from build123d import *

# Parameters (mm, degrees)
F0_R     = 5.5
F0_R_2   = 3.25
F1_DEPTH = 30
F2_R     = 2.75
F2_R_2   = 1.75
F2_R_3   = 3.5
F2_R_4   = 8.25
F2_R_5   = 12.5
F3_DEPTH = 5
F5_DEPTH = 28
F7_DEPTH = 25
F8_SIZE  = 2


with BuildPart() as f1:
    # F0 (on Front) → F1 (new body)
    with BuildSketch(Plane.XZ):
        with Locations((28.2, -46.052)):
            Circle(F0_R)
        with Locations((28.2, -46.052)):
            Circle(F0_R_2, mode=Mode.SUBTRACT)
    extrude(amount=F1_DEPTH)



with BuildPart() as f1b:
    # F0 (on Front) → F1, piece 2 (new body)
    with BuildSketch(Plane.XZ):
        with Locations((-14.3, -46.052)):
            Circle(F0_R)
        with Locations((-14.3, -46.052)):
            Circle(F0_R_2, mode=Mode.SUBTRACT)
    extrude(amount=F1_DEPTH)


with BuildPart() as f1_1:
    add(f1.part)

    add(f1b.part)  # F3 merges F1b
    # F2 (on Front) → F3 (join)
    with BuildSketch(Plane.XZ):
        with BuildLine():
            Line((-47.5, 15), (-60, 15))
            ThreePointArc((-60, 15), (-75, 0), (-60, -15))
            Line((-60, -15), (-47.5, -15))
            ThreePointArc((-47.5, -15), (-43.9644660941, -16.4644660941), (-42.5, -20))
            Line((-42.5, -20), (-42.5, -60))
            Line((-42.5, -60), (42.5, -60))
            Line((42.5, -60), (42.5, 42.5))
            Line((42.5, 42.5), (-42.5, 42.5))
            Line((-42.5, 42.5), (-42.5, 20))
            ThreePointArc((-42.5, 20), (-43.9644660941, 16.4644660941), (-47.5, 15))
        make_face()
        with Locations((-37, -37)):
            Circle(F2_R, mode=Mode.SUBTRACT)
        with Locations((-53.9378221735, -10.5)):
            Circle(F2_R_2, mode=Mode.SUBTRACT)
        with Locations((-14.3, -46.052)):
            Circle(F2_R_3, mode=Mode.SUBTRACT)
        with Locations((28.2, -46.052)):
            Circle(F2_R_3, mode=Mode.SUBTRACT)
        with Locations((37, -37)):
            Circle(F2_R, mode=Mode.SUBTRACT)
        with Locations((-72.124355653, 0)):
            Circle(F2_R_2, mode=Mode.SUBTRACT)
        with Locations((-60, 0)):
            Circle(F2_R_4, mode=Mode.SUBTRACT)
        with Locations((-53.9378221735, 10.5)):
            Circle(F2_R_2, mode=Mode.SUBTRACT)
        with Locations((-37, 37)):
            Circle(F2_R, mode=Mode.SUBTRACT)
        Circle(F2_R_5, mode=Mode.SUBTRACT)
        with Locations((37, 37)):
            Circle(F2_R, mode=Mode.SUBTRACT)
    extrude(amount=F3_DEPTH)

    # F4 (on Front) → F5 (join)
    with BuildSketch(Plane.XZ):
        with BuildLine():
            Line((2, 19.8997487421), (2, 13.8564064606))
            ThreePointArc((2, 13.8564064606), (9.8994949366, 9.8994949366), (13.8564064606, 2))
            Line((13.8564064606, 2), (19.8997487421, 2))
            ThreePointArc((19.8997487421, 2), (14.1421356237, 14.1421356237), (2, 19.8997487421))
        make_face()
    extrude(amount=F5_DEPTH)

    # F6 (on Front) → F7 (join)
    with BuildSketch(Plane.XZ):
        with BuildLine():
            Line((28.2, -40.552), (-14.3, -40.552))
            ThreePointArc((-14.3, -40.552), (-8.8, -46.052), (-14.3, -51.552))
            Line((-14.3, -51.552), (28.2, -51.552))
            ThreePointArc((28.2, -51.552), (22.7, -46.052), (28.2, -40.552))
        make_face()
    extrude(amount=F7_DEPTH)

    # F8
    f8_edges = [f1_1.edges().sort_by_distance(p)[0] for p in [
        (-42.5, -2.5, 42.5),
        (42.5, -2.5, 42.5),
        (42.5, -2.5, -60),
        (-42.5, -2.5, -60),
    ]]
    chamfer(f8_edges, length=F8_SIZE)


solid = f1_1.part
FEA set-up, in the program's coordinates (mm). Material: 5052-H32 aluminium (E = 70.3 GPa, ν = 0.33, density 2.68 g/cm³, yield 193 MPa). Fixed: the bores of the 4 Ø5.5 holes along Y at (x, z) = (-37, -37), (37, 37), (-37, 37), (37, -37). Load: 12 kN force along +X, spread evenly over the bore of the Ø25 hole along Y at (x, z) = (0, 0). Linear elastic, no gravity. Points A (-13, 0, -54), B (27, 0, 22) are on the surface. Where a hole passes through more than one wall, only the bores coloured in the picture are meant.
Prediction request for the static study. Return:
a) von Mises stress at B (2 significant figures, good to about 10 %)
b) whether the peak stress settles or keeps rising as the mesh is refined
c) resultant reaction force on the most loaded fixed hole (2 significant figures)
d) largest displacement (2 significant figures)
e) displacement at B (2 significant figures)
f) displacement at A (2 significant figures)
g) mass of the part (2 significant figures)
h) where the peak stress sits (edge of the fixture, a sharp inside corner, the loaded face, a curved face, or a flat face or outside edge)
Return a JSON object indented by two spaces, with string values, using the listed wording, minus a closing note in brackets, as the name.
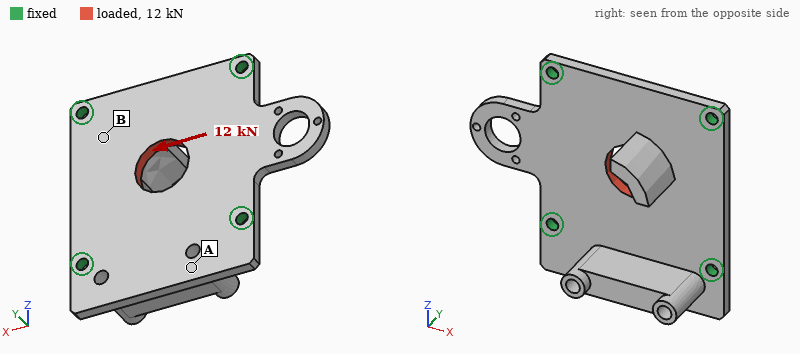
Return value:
{
  "von Mises stress at B": "30 MPa",
  "whether the peak stress settles or keeps rising as the mesh is refined": "keeps rising",
  "resultant reaction force on the most loaded fixed hole": "3.4 kN",
  "largest displacement": "27 µm",
  "displacement at B": "13 µm",
  "displacement at A": "5.0 µm",
  "mass of the part": "150 g",
  "where the peak stress sits": "edge of the fixture"
}
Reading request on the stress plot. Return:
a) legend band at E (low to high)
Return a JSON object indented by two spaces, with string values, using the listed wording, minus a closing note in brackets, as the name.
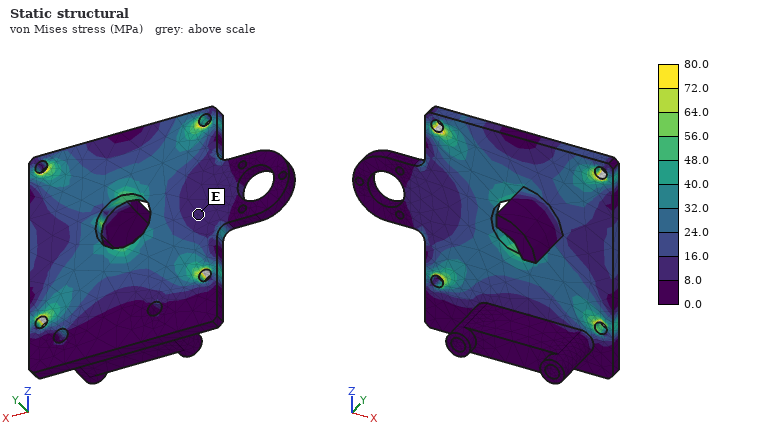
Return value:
{
  "legend band at E": "8.0 to 16.0 MPa"
}
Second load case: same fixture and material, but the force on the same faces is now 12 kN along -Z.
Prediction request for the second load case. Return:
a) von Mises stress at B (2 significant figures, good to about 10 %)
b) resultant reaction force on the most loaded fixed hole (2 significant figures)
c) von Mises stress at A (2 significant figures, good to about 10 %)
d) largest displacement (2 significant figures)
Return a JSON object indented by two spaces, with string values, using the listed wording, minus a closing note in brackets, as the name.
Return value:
{
  "von Mises stress at B": "28 MPa",
  "resultant reaction force on the most loaded fixed hole": "3.4 kN",
  "von Mises stress at A": "16 MPa",
  "largest displacement": "27 µm"
}
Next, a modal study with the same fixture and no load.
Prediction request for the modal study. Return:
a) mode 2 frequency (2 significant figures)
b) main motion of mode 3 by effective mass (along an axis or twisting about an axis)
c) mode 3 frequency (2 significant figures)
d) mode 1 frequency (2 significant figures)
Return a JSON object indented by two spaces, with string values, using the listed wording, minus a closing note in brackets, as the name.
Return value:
{
  "mode 2 frequency": "2700 Hz",
  "main motion of mode 3 by effective mass": "along Y",
  "mode 3 frequency": "3500 Hz",
  "mode 1 frequency": "2300 Hz"
}
